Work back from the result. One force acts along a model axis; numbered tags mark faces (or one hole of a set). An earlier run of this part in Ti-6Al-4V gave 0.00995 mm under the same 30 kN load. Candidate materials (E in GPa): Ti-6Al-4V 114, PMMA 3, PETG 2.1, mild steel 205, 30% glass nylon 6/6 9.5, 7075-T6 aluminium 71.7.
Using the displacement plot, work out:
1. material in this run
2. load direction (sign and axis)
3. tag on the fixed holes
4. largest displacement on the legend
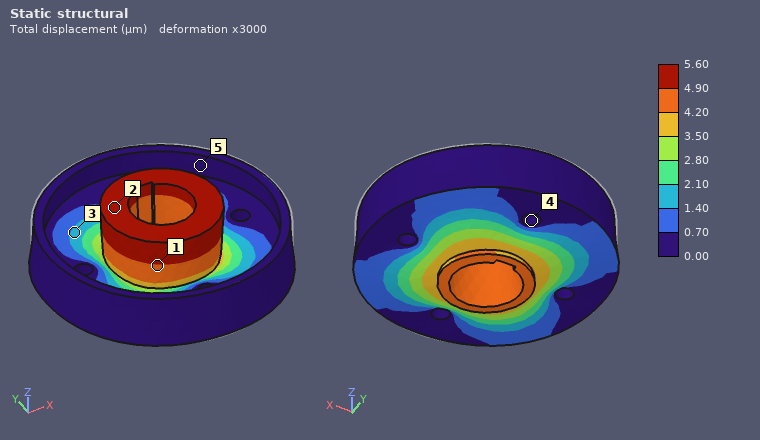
mild steel
-Z
4
5.60 µm
